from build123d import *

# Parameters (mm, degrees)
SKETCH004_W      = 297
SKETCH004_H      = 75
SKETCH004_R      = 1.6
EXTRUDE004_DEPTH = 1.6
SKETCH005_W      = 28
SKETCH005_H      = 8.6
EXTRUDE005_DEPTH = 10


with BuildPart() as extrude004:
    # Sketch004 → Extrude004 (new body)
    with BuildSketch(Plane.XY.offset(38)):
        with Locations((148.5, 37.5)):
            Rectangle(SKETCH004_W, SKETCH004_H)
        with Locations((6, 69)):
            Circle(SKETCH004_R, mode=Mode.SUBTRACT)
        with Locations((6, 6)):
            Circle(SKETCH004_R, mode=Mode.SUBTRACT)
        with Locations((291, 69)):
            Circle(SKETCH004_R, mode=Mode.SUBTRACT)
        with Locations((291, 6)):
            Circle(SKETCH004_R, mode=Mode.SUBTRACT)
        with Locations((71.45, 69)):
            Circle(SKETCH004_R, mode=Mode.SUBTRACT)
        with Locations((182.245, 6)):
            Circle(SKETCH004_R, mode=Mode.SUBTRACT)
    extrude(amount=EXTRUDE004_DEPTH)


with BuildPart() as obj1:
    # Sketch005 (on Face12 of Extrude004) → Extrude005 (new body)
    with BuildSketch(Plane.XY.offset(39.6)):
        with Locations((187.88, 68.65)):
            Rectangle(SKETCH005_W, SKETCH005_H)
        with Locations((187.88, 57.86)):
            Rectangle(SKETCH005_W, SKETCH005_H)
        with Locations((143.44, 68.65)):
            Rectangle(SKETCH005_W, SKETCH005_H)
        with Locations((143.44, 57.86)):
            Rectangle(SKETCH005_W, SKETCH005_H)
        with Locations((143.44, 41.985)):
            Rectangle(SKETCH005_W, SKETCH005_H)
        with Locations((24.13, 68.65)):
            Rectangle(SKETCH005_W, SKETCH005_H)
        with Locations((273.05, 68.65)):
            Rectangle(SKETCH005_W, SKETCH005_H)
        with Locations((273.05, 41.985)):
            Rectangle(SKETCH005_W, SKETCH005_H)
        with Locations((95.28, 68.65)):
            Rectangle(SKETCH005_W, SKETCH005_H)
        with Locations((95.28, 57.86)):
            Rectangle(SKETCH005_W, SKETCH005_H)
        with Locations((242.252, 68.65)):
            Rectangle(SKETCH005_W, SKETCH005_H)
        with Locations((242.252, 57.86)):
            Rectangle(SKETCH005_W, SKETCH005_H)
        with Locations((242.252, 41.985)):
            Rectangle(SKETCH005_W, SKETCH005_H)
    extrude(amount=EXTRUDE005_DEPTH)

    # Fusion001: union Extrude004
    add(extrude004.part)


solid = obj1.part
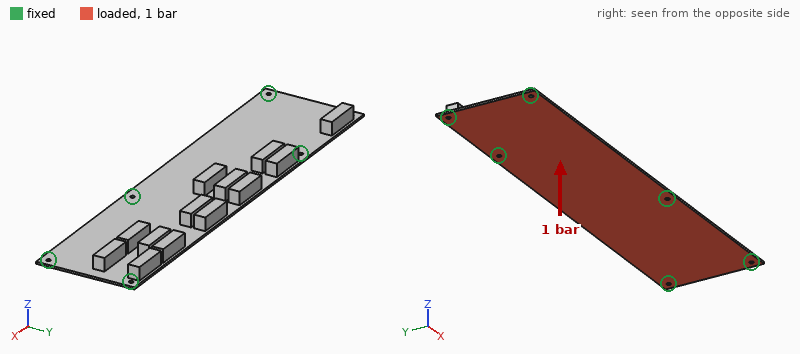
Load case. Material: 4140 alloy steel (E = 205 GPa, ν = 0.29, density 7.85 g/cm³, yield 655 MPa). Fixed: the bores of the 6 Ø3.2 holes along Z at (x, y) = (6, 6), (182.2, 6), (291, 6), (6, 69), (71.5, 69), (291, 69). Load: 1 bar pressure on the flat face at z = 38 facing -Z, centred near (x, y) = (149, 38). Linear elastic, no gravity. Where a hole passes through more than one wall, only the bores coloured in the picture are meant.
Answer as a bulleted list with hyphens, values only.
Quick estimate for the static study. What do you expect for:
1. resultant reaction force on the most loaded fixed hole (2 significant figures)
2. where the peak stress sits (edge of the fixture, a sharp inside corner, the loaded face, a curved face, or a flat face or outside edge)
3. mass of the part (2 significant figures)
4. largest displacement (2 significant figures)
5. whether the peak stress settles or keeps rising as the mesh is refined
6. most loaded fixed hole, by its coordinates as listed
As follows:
- 810 N
- edge of the fixture
- 520 g
- 1.5 mm
- keeps rising
- (182.2, 6)
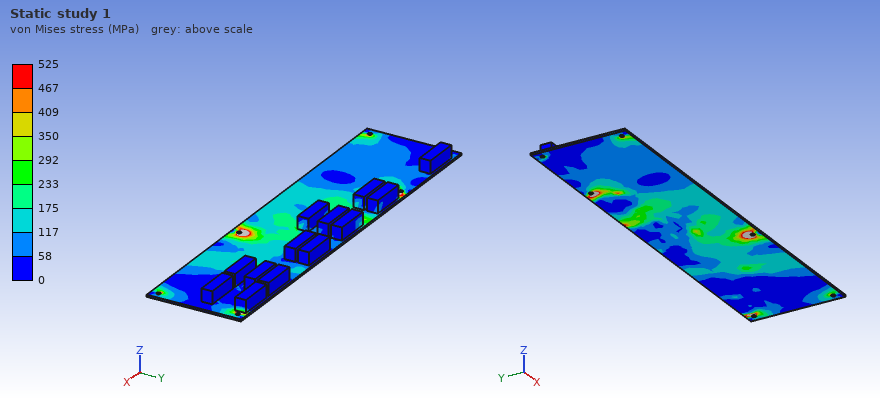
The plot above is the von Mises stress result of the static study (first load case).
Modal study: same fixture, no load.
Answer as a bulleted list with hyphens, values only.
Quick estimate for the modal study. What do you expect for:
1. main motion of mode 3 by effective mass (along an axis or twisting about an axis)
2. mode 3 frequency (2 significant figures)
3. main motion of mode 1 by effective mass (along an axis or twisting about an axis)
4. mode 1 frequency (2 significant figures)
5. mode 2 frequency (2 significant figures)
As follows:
- along Z
- 510 Hz
- along Z
- 270 Hz
- 380 Hz
